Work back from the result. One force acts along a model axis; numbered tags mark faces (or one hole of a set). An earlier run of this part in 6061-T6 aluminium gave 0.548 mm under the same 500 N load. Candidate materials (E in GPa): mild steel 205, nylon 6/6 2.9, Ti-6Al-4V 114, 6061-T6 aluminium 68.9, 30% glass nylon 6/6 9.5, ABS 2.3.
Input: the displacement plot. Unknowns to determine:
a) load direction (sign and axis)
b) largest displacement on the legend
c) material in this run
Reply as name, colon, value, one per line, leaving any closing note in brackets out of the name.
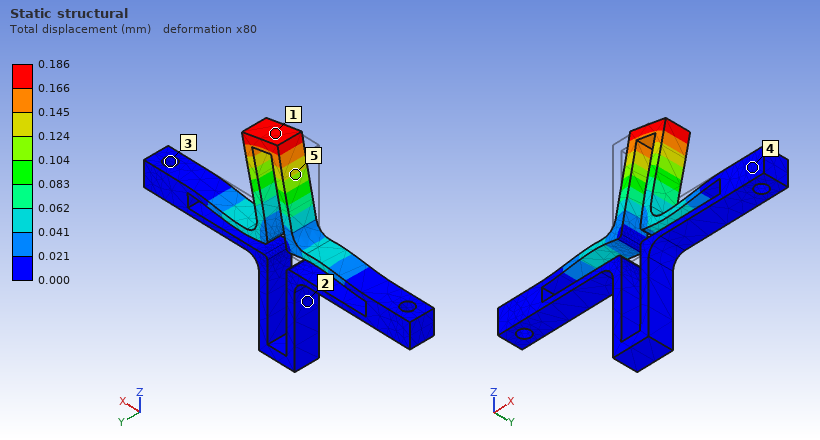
load direction: +X
largest displacement on the legend: 0.186 mm
material in this run: mild steel
